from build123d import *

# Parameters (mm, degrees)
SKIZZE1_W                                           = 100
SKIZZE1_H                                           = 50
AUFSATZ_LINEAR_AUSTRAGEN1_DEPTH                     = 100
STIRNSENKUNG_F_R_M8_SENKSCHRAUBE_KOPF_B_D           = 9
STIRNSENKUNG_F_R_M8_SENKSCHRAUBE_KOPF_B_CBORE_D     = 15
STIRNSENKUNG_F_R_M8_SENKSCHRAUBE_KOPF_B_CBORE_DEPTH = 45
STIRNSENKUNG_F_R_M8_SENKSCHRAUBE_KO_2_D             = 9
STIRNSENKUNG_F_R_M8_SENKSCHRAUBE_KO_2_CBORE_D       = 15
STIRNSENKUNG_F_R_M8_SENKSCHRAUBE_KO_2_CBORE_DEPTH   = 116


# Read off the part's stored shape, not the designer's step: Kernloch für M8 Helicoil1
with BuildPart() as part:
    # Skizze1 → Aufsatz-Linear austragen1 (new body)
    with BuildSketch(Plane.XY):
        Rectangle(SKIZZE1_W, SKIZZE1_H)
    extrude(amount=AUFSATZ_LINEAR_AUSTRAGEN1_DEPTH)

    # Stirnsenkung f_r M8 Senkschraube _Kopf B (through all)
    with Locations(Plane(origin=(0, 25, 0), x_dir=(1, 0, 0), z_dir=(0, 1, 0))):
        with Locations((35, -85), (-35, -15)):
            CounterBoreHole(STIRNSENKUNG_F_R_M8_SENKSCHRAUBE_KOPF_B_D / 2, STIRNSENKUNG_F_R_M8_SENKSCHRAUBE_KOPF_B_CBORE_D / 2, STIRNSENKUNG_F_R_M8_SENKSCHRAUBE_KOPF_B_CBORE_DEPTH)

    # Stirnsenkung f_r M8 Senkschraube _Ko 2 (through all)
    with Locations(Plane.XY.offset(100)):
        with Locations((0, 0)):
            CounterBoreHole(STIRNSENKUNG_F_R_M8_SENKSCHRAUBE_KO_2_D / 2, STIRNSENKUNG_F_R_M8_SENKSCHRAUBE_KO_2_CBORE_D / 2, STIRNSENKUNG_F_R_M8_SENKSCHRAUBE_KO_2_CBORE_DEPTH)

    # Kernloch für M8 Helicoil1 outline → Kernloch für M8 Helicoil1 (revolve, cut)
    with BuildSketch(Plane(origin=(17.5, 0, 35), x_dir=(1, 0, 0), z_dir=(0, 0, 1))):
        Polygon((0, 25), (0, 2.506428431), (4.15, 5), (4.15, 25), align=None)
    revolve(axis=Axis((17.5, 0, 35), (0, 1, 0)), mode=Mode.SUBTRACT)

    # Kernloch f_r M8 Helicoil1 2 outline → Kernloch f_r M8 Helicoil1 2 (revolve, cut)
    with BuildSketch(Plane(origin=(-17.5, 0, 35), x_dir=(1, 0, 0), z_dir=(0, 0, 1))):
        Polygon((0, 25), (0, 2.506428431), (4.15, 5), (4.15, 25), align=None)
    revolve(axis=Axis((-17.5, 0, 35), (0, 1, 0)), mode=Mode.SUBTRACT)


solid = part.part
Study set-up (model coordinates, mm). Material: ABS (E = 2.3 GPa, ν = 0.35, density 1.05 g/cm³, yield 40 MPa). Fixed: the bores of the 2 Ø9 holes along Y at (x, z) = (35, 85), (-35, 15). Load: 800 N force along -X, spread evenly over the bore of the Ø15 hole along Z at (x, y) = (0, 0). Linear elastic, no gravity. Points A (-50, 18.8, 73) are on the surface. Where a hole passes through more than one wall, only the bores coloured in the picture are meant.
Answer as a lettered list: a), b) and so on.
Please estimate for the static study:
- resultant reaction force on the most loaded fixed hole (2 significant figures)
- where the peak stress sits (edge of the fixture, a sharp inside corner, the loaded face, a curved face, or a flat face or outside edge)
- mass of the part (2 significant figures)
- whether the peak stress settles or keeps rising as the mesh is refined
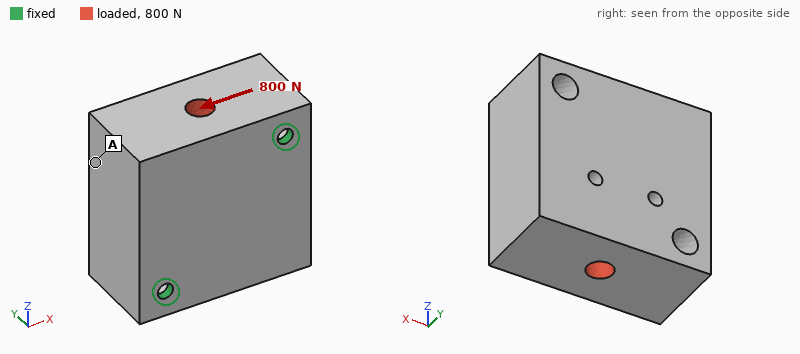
a) 420 N
b) edge of the fixture
c) 490 g
d) keeps rising
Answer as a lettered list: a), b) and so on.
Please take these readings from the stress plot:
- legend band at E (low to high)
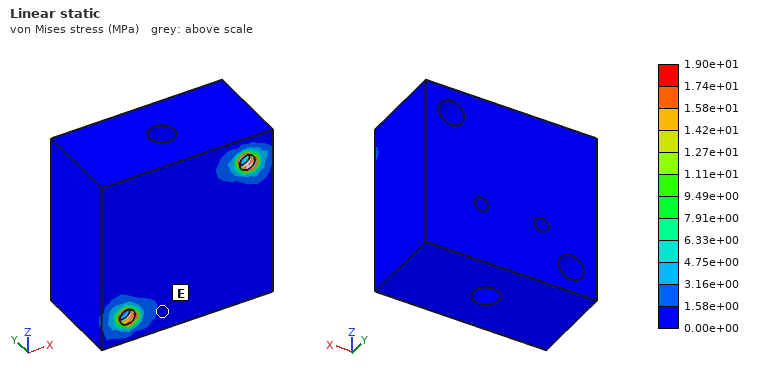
a) 0.00e+00 to 1.58e+00 MPa
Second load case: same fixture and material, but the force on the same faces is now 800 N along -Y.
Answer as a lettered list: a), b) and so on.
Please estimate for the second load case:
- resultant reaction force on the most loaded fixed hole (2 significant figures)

a) 430 N
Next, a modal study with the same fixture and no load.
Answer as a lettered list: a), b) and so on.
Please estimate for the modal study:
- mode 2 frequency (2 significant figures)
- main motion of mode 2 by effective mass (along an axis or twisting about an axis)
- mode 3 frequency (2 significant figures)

a) 1200 Hz
b) along Y
c) 1400 Hz
